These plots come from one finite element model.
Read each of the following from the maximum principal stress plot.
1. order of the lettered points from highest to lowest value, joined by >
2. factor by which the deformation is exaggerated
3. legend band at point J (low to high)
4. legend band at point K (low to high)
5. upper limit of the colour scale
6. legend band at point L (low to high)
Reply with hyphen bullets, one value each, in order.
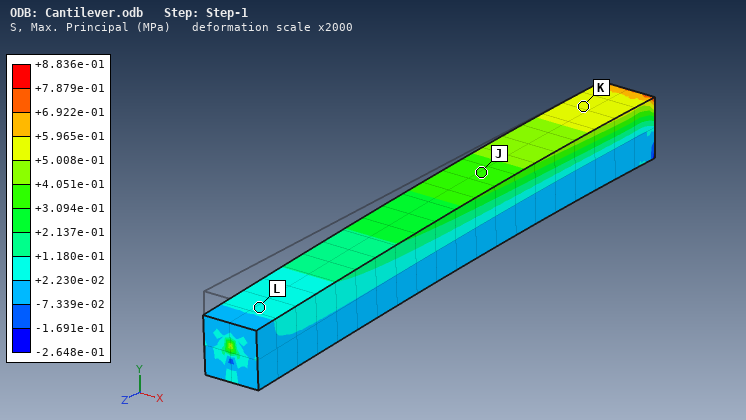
- K > J > L
- 2000
- +3.094e-01 to +4.051e-01 MPa
- +5.008e-01 to +5.965e-01 MPa
- +8.836e-01 MPa
- +2.230e-02 to +1.180e-01 MPa
